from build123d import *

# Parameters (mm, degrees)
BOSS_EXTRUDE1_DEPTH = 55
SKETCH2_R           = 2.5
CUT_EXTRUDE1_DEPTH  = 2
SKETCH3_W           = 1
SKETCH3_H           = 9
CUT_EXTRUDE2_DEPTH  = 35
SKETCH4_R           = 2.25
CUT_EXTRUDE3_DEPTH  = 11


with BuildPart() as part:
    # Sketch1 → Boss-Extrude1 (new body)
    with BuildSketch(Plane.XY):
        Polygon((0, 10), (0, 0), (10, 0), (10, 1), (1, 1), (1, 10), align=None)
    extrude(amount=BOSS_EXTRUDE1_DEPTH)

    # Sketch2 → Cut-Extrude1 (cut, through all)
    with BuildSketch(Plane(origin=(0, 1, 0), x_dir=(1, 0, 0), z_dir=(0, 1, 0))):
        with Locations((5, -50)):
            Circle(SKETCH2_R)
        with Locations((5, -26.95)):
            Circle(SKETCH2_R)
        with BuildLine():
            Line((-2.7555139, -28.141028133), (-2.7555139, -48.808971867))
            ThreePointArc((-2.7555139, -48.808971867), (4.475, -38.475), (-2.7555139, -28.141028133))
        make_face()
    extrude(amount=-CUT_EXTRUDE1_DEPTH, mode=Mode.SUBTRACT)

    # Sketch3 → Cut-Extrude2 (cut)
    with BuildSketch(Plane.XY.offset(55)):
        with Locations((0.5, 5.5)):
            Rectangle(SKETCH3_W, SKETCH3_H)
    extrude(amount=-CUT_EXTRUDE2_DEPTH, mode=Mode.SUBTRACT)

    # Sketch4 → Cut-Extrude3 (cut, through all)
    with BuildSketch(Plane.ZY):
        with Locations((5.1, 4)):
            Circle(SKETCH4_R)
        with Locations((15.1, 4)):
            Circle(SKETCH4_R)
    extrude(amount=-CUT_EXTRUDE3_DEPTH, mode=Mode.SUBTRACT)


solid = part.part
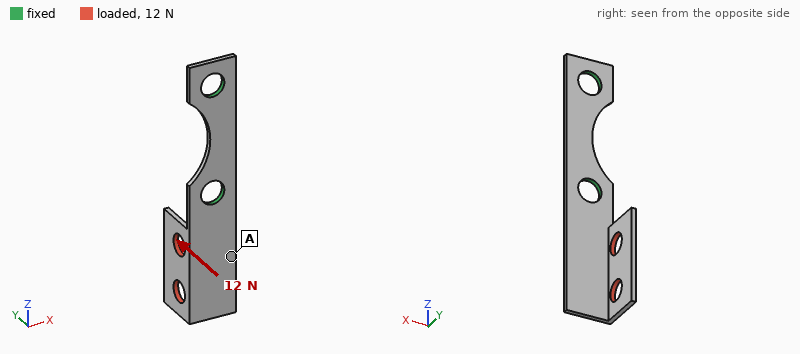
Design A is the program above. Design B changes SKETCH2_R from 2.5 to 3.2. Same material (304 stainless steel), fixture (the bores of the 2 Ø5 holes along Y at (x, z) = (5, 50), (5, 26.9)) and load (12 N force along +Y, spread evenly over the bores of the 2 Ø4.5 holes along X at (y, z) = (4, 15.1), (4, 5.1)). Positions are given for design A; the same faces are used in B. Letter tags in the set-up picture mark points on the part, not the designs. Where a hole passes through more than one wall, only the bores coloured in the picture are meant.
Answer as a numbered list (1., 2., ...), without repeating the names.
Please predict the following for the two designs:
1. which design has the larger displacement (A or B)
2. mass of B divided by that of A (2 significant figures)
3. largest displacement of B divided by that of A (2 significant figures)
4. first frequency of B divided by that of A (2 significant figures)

1. A
2. 0.96
3. 0.86
4. 1.1
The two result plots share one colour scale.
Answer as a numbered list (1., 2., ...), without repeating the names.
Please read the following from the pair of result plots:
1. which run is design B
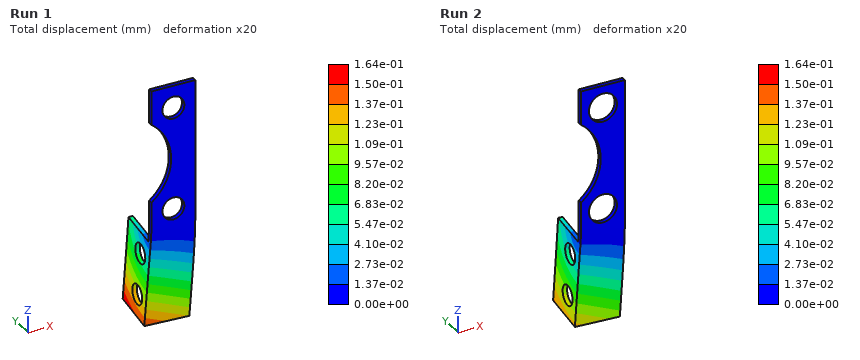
1. Run 2
